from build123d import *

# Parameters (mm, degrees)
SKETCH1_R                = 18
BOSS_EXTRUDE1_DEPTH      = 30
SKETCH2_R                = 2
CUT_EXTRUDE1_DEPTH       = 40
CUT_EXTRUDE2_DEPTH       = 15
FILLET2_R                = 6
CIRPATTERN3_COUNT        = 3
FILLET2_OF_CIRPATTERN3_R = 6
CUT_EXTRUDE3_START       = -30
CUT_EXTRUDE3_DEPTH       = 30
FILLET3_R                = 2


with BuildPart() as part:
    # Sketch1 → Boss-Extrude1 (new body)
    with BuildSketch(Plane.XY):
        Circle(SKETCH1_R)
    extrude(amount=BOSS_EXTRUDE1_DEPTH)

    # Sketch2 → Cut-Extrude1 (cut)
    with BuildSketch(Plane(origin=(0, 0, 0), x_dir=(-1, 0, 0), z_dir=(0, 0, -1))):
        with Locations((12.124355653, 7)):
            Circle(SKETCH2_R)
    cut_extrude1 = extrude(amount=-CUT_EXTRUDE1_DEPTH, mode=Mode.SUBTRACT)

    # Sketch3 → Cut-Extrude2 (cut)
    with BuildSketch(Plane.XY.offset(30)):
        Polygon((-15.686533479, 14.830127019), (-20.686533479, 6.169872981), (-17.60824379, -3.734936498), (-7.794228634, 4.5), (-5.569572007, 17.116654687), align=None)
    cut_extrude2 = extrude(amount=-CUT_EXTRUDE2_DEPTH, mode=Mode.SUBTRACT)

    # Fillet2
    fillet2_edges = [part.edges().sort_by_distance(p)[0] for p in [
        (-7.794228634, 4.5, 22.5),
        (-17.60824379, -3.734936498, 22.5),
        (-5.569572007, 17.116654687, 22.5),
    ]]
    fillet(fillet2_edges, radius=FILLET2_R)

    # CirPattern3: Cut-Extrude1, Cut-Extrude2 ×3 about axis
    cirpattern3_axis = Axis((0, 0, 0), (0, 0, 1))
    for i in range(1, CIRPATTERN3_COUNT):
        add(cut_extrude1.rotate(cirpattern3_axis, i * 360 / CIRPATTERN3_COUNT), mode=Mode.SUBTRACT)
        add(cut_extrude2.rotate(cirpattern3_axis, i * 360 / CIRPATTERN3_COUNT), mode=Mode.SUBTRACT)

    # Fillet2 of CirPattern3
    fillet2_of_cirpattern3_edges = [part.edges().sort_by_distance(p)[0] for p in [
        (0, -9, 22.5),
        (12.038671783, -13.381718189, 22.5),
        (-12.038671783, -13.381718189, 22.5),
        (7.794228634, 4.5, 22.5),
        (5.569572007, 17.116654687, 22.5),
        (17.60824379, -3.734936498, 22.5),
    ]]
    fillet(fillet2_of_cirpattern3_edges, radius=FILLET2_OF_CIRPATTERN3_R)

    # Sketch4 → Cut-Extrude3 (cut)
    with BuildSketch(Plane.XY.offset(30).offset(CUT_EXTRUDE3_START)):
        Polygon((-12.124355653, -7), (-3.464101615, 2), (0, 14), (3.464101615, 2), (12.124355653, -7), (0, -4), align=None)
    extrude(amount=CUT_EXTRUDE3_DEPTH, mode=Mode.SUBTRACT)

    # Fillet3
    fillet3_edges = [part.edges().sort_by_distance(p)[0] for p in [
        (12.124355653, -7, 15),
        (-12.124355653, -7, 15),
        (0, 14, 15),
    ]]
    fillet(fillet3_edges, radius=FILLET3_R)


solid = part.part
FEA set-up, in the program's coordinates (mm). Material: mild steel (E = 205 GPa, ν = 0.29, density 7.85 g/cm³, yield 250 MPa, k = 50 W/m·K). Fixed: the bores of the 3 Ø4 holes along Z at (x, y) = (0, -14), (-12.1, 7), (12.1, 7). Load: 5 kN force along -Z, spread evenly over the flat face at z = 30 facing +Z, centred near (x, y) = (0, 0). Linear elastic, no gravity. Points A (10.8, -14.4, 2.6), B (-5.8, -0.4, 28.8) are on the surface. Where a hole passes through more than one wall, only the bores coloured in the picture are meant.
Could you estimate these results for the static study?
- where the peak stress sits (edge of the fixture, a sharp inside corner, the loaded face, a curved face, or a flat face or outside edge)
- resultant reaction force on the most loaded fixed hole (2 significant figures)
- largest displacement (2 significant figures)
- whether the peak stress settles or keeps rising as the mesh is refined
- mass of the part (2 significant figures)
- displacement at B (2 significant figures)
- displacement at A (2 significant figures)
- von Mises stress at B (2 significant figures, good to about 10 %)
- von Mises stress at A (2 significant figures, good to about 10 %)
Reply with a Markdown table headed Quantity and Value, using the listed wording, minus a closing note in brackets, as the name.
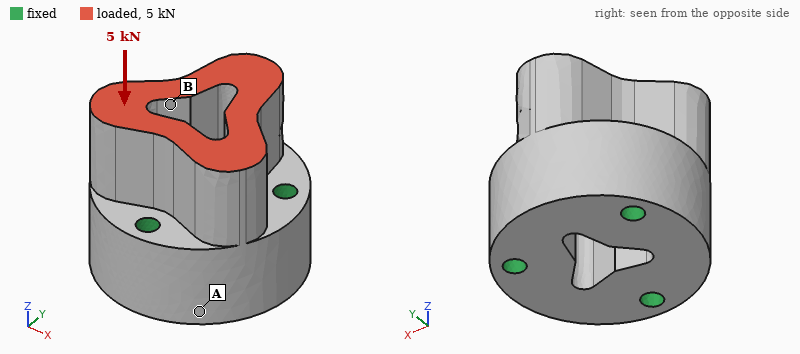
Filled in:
| Quantity | Value |
|---|---|
| where the peak stress sits | edge of the fixture |
| resultant reaction force on the most loaded fixed hole | 1.7 kN |
| largest displacement | 1.6 µm |
| whether the peak stress settles or keeps rising as the mesh is refined | keeps rising |
| mass of the part | 160 g |
| displacement at B | 1.4 µm |
| displacement at A | 0.56 µm |
| von Mises stress at B | 11 MPa |
| von Mises stress at A | 4.0 MPa |
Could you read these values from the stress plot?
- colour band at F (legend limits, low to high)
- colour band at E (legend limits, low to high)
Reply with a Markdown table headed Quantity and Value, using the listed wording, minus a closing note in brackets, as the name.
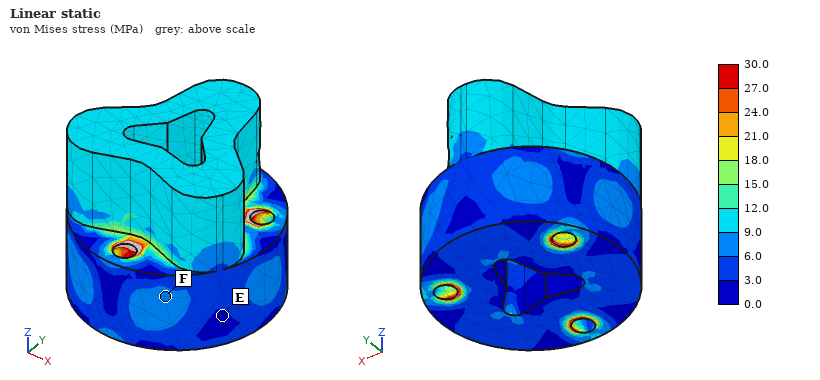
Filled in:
| Quantity | Value |
|---|---|
| colour band at F | 6.0 to 9.0 MPa |
| colour band at E | 0.0 to 3.0 MPa |
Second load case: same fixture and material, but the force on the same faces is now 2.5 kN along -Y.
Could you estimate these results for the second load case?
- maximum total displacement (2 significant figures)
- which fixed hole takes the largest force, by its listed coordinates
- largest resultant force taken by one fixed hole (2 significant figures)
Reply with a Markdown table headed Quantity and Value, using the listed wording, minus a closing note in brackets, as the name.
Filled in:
| Quantity | Value |
|---|---|
| maximum total displacement | 6.7 µm |
| which fixed hole takes the largest force, by its listed coordinates | (0, -14) |
| largest resultant force taken by one fixed hole | 1.9 kN |
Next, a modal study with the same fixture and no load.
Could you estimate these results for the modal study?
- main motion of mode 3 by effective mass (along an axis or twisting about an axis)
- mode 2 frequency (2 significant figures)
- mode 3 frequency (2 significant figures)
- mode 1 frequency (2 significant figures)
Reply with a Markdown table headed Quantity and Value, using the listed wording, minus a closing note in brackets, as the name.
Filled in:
| Quantity | Value |
|---|---|
| main motion of mode 3 by effective mass | twisting about Z |
| mode 2 frequency | 22 kHz |
| mode 3 frequency | 34 kHz |
| mode 1 frequency | 22 kHz |
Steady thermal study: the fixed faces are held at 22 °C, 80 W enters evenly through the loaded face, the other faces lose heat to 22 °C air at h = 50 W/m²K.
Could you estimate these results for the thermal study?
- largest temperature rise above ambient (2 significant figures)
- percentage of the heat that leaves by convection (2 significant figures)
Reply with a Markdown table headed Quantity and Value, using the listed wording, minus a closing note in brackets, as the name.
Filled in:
| Quantity | Value |
|---|---|
| largest temperature rise above ambient | 69 K |
| percentage of the heat that leaves by convection | 8.2 % |
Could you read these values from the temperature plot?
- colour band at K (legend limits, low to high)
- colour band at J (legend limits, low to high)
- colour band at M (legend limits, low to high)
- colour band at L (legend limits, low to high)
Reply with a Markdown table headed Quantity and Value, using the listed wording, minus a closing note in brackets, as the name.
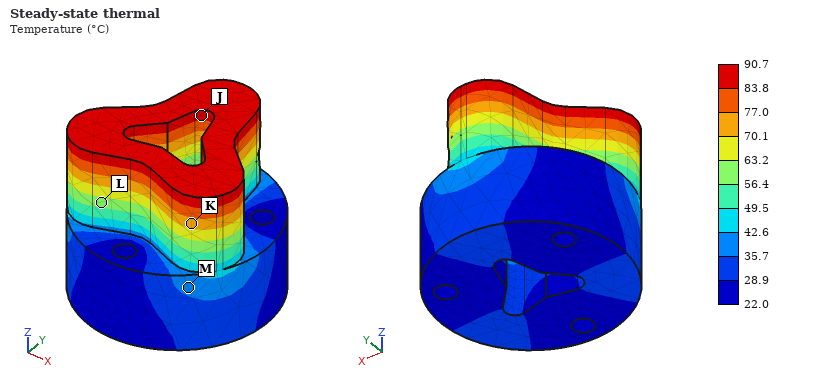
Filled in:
| Quantity | Value |
|---|---|
| colour band at K | 70.1 to 77.0 °C |
| colour band at J | 83.8 to 90.7 °C |
| colour band at M | 35.7 to 42.6 °C |
| colour band at L | 56.4 to 63.2 °C |
